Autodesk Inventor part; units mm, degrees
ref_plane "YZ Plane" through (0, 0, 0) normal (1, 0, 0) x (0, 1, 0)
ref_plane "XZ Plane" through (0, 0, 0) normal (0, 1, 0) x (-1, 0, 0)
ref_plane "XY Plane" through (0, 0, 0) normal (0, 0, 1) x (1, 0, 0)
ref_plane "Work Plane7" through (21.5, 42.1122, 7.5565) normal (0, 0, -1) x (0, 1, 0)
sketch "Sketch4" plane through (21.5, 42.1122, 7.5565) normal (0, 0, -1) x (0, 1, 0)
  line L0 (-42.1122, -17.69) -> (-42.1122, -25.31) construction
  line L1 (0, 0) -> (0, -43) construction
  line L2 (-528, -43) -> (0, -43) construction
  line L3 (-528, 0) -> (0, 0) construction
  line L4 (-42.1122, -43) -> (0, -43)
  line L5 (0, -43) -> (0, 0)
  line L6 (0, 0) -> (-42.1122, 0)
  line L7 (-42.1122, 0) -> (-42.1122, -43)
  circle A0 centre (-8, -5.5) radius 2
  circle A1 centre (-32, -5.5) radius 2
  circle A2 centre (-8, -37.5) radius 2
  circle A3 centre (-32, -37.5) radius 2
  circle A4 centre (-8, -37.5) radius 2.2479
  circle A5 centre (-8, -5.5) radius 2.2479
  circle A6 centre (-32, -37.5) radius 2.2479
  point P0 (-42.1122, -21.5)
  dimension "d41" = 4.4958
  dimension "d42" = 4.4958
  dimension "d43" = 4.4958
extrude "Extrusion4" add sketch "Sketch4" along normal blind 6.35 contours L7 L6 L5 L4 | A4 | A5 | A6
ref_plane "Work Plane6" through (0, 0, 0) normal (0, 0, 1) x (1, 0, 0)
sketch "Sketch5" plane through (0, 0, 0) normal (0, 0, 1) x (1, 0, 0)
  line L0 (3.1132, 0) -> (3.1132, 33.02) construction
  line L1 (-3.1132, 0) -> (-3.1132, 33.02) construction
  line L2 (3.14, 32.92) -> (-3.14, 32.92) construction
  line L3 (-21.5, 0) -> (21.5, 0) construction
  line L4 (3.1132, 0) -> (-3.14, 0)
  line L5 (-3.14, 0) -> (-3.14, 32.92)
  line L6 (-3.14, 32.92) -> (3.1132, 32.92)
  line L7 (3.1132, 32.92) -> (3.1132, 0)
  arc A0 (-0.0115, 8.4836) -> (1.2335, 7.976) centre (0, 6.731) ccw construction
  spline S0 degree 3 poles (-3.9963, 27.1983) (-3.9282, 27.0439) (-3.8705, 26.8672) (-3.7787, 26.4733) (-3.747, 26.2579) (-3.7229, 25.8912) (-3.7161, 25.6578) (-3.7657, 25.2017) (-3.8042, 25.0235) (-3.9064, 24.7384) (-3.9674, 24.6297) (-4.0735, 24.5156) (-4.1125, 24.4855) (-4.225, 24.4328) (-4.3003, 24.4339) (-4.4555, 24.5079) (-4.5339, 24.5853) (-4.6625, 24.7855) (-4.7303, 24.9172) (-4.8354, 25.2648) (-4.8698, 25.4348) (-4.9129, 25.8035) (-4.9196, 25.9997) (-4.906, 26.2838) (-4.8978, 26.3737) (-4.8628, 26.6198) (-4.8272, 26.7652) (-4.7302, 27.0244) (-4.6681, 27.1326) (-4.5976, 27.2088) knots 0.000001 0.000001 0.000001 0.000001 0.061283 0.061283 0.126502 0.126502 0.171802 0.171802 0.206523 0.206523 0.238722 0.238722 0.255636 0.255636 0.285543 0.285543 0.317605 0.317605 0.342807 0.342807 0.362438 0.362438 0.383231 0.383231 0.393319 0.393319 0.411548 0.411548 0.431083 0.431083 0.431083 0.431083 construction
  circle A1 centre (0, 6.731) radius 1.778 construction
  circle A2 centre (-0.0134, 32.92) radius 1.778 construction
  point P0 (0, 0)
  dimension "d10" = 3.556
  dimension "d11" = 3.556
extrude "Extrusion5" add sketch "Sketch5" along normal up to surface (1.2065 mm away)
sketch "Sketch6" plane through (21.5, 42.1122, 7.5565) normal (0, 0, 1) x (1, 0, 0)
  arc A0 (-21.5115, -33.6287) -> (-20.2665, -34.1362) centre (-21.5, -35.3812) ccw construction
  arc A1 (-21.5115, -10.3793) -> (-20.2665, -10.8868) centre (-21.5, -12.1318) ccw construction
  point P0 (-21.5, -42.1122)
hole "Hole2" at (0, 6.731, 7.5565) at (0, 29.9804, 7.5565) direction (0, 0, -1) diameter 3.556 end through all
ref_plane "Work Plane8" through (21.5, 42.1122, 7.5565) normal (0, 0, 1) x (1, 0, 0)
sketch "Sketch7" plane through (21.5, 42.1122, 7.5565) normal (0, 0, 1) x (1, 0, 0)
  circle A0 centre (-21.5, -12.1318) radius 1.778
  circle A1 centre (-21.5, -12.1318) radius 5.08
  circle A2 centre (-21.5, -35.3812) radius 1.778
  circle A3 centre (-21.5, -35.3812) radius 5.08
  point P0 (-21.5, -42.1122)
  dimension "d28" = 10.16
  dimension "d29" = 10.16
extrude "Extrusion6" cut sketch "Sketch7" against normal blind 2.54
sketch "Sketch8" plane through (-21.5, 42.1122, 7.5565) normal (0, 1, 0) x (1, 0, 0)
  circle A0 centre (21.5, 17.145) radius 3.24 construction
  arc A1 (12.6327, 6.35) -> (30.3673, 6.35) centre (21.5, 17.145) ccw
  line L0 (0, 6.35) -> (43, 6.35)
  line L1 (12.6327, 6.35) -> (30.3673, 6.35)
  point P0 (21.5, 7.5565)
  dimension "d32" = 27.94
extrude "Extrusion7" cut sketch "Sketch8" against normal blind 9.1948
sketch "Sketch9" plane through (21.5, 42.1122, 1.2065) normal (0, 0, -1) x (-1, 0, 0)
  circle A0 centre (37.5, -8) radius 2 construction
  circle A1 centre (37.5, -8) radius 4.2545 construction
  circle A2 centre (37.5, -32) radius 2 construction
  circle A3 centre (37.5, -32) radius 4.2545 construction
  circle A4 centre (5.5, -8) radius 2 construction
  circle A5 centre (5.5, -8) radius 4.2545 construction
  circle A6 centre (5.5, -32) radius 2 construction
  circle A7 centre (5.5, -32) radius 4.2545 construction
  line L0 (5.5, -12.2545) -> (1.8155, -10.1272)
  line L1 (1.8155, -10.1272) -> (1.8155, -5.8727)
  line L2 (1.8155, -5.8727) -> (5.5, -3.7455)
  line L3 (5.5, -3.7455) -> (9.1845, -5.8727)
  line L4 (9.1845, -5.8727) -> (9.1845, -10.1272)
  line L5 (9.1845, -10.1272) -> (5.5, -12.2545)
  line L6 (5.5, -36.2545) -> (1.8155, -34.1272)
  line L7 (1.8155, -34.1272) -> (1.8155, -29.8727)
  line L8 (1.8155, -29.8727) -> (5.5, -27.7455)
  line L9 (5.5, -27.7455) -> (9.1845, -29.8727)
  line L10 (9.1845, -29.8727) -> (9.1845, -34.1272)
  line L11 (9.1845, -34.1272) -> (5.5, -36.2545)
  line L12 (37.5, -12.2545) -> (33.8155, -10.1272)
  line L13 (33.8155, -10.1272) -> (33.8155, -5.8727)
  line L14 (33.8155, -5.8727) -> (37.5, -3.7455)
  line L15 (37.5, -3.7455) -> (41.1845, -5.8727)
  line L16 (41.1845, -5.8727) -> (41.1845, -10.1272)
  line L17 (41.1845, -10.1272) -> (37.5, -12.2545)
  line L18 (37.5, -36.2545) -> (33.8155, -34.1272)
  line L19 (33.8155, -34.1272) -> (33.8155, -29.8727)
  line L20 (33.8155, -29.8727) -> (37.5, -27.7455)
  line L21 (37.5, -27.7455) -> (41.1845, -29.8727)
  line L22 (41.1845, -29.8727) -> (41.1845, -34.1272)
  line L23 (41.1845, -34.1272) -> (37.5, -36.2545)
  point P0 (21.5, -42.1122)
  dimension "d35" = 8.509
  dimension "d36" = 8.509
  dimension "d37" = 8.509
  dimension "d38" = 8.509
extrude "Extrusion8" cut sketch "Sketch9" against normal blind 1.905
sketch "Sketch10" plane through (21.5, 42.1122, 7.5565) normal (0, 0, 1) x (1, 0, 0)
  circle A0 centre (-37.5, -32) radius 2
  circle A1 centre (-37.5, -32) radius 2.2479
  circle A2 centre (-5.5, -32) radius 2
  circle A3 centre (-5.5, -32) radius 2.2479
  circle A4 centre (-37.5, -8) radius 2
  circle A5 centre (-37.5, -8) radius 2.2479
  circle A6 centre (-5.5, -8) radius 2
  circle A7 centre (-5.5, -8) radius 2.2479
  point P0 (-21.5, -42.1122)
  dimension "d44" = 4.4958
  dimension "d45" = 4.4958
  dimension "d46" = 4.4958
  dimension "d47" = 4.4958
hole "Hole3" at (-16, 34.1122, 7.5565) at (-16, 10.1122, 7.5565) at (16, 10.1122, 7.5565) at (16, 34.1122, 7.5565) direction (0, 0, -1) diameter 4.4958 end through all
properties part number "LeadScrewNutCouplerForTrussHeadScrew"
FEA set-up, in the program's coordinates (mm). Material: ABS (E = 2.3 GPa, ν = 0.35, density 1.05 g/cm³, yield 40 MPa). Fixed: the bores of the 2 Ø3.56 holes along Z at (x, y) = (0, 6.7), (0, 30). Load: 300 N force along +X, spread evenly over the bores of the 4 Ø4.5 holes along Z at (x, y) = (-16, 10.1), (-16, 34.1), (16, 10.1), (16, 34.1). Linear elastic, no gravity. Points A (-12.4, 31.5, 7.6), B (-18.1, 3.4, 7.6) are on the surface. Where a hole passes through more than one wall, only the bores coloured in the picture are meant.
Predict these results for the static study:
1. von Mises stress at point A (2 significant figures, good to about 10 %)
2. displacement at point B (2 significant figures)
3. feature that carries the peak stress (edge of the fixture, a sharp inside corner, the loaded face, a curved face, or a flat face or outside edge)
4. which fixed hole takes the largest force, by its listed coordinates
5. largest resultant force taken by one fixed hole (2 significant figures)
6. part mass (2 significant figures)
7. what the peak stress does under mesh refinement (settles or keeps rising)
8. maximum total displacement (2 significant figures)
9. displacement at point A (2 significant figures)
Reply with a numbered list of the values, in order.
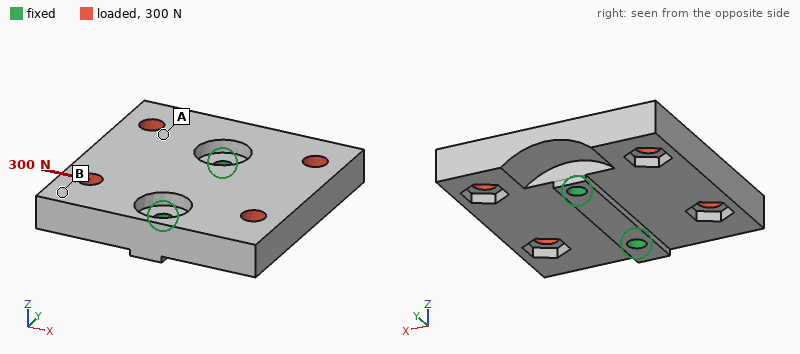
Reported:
1. 1.5 MPa
2. 0.068 mm
3. edge of the fixture
4. (0, 30)
5. 200 N
6. 11 g
7. keeps rising
8. 0.10 mm
9. 0.059 mm
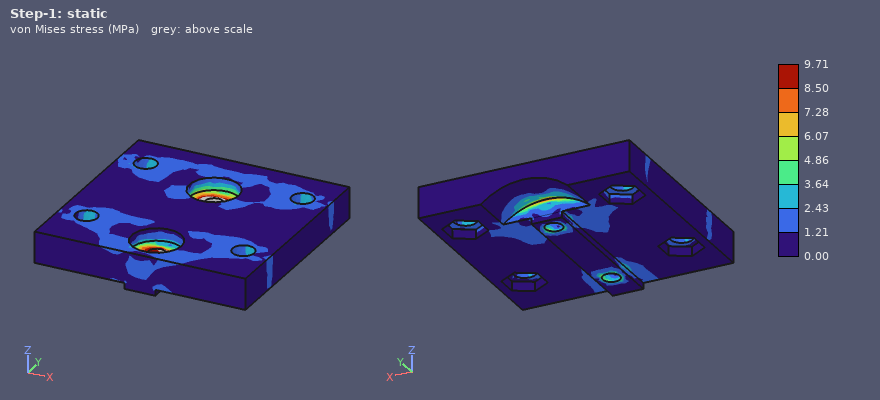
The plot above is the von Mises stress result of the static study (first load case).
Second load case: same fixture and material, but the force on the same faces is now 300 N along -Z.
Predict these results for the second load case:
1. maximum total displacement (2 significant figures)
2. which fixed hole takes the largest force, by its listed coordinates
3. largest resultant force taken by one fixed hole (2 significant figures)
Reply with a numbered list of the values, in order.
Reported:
1. 0.29 mm
2. (0, 30)
3. 200 N
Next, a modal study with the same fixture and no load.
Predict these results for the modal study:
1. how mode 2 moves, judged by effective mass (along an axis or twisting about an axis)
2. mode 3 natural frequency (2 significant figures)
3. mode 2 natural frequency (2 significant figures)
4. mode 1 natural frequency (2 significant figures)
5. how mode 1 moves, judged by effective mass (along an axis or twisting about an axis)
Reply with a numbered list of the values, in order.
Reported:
1. along Z
2. 3300 Hz
3. 2800 Hz
4. 1700 Hz
5. twisting about Y
